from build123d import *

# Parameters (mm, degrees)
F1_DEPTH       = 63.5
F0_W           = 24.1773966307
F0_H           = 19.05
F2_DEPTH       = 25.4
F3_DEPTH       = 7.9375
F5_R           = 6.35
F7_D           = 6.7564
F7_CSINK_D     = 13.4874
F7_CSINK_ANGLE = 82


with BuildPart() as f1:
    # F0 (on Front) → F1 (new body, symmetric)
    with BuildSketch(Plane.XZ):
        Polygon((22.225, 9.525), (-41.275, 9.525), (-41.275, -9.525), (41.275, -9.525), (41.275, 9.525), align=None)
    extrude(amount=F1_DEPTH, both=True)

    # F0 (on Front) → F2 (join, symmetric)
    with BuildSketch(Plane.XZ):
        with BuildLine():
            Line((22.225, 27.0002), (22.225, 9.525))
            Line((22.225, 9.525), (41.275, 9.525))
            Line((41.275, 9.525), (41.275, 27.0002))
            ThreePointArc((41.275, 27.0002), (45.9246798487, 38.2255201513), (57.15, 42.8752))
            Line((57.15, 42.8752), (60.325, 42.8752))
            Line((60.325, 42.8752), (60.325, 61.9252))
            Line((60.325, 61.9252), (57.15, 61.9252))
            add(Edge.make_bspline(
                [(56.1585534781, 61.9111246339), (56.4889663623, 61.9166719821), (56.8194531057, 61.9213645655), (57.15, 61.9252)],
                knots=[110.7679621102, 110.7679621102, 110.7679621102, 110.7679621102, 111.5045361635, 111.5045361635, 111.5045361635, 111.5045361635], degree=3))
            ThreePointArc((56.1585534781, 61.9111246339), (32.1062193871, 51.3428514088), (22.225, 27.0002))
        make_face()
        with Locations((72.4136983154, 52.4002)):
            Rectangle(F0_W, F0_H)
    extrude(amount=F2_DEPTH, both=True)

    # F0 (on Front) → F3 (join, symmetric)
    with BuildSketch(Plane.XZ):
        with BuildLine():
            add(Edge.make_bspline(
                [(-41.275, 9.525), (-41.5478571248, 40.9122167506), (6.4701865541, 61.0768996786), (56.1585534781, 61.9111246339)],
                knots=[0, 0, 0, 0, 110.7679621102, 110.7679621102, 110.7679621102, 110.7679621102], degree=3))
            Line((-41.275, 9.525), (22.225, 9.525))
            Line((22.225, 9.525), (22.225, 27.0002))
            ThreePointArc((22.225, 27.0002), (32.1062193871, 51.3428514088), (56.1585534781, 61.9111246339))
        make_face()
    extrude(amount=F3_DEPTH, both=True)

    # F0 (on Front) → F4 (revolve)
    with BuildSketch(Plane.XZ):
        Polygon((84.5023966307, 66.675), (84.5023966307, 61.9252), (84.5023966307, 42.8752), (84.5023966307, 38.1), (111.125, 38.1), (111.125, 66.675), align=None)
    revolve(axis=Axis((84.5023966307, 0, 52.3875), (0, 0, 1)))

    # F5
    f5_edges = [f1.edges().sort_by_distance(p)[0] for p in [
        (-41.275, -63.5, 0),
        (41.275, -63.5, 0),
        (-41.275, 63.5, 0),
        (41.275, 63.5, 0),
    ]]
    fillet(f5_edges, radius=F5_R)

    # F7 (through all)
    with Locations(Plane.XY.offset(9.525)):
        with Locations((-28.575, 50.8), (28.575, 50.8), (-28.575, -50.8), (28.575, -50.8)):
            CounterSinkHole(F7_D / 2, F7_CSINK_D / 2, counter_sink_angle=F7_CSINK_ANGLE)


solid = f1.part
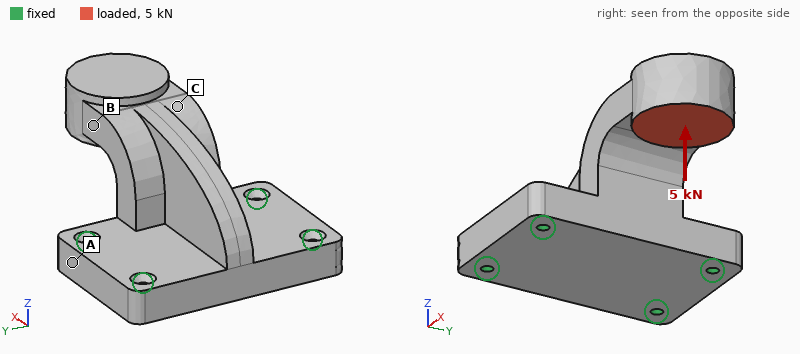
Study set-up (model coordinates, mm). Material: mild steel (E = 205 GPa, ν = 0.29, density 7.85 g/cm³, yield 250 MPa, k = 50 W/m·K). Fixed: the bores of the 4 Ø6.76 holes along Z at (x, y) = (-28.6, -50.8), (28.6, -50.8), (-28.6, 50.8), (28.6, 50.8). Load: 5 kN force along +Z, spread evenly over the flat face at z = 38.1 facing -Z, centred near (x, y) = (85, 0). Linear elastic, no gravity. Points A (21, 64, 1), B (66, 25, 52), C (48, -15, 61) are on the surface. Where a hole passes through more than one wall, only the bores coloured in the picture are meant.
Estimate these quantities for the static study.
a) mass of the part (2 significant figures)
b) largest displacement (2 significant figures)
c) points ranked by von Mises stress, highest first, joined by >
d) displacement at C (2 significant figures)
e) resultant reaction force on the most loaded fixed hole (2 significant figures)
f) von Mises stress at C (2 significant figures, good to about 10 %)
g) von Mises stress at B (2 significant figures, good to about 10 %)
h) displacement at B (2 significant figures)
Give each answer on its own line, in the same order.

2.8 kg
0.12 mm
C > B > A
0.040 mm
5.0 kN
35 MPa
20 MPa
0.051 mm
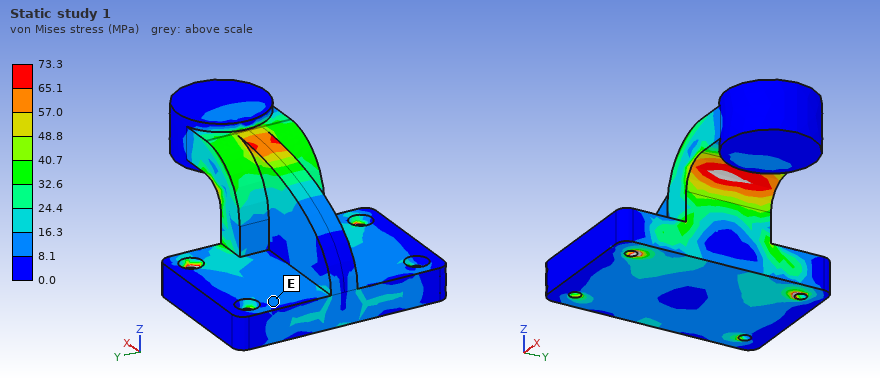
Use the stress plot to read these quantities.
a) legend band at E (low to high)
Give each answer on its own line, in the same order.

8.1 to 16.3 MPa
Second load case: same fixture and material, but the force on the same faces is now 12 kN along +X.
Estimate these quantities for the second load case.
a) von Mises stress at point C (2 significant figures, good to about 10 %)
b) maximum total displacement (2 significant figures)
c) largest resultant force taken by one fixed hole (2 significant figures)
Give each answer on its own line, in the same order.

28 MPa
36 µm
5.6 kN
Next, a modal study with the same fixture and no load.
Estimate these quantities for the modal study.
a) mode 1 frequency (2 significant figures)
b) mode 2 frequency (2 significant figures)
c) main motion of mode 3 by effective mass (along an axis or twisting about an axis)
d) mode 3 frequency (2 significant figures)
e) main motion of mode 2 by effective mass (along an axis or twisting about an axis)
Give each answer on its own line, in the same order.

1600 Hz
1900 Hz
along X
3800 Hz
along Y
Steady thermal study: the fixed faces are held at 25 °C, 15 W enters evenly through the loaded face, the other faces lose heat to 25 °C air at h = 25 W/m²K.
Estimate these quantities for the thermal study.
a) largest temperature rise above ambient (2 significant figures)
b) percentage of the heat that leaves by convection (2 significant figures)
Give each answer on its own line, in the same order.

21 K
41 %
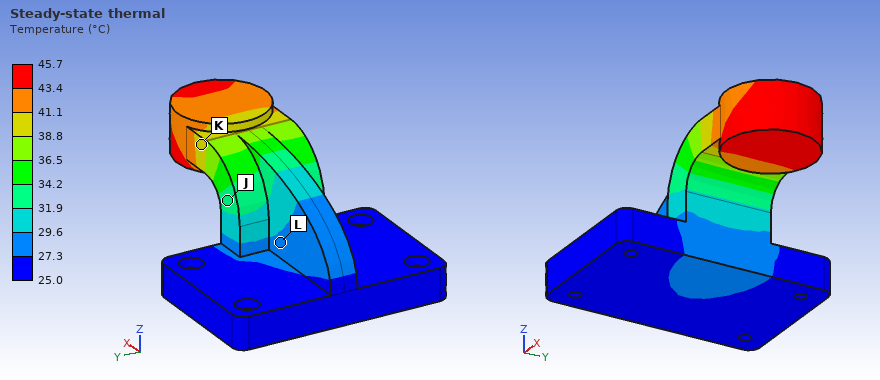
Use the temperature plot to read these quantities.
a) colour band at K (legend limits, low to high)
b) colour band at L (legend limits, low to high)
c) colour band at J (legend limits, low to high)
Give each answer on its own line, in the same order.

38.8 to 41.1 °C
27.3 to 29.6 °C
31.9 to 34.2 °C
